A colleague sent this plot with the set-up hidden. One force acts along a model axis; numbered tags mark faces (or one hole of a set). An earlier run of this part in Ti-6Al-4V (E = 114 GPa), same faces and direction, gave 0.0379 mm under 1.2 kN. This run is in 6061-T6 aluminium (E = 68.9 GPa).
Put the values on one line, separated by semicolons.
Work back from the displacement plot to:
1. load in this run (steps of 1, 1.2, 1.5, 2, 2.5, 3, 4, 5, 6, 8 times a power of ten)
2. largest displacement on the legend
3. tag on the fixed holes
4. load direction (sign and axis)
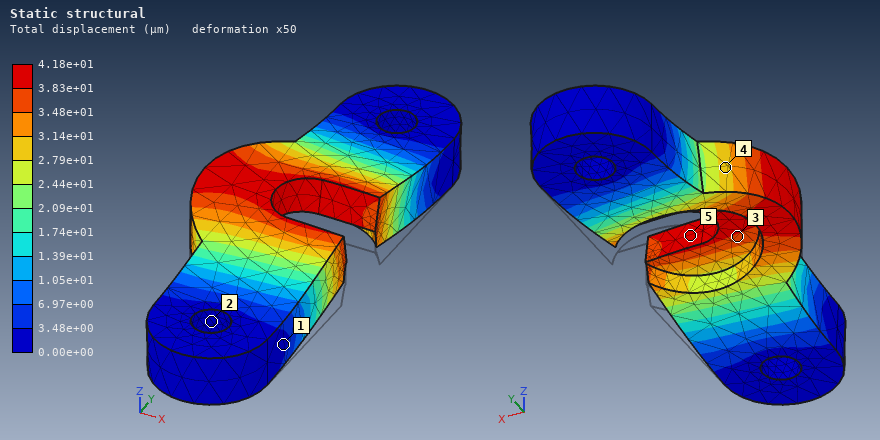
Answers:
800 N; 4.18e+01 µm; 2; +Z
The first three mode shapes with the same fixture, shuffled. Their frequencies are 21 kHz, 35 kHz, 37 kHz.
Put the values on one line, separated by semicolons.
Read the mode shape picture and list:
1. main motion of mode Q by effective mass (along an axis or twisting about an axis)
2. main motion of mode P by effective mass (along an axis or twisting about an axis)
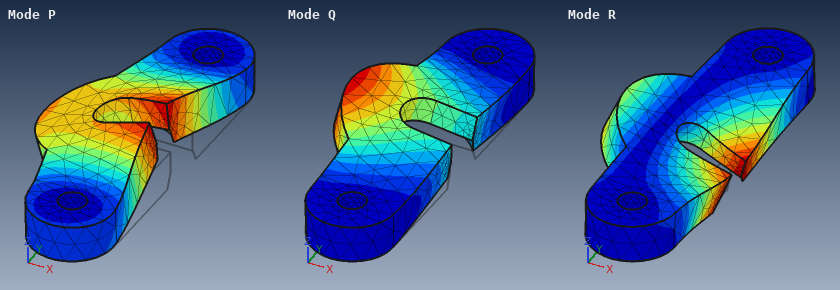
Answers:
along Z; along X
